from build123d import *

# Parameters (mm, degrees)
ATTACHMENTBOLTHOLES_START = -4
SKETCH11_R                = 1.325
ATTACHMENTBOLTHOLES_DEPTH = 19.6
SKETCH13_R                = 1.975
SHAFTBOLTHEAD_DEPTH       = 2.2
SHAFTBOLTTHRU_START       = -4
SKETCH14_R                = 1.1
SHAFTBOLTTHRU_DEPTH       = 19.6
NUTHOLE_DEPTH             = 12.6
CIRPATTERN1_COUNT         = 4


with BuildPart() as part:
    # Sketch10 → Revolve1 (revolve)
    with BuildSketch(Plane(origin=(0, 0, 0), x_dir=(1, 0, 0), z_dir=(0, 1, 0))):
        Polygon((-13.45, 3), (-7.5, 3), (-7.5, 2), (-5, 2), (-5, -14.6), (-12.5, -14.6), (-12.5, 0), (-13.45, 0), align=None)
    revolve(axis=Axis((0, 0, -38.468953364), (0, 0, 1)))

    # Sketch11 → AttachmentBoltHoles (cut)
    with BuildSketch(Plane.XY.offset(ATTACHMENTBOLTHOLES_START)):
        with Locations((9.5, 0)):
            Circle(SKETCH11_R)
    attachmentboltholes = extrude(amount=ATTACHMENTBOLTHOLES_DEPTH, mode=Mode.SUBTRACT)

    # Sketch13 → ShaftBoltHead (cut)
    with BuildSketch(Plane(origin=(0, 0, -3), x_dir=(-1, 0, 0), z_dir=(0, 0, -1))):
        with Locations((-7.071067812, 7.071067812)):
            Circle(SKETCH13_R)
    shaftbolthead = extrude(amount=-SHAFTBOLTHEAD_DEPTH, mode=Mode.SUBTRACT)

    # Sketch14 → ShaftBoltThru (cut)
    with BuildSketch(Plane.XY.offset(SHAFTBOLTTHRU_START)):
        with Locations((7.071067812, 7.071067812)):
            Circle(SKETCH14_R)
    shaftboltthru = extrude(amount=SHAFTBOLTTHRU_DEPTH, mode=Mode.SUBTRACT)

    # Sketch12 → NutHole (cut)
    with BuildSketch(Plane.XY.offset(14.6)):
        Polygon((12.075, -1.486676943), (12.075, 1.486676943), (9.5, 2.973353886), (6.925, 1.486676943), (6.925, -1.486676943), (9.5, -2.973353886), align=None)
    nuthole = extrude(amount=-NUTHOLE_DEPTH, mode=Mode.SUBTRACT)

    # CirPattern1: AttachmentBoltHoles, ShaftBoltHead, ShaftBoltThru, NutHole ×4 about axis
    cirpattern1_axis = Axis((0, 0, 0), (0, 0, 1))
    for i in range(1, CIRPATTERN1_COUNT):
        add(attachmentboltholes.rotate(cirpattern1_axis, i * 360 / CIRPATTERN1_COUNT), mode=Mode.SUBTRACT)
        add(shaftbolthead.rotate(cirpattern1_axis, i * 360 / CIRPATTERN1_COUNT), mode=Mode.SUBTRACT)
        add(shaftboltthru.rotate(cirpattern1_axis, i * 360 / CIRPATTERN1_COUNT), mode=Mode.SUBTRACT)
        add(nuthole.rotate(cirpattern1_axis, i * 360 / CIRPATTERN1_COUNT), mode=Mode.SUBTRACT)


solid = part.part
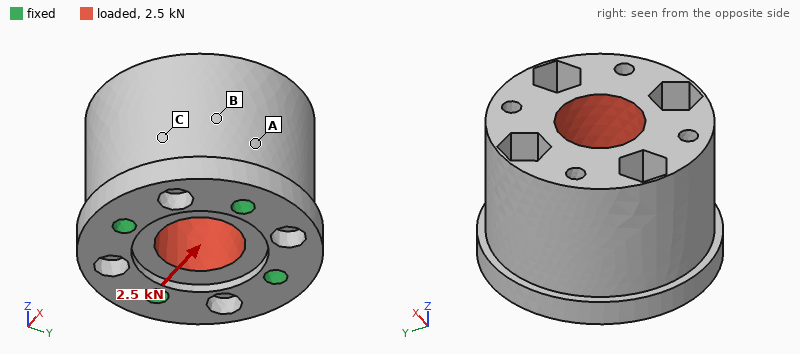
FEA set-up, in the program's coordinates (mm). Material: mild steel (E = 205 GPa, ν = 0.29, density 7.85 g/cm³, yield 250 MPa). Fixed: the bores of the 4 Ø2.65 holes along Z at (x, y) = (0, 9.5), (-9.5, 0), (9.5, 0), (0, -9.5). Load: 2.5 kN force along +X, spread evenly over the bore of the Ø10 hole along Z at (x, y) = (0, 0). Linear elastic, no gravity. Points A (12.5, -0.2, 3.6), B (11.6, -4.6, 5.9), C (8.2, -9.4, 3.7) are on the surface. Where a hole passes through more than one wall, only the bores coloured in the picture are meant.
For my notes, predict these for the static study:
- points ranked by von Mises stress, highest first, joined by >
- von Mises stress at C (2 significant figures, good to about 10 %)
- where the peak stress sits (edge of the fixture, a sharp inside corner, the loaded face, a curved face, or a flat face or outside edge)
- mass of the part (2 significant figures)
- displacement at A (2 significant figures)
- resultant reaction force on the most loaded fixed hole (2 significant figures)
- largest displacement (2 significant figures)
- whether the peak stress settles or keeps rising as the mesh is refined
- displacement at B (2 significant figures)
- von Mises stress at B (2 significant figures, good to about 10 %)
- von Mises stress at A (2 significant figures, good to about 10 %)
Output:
A > B > C
5.3 MPa
edge of the fixture
45 g
0.93 µm
970 N
3.0 µm
keeps rising
1.7 µm
9.6 MPa
25 MPa
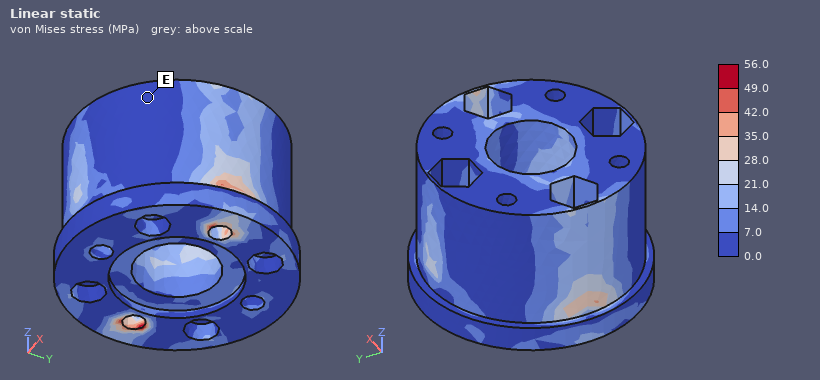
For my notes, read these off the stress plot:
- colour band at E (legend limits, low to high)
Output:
0.0 to 7.0 MPa
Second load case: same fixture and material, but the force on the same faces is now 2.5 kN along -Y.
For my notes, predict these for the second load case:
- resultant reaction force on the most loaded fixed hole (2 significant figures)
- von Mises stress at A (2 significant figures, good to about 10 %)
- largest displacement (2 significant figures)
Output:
970 N
21 MPa
3.0 µm
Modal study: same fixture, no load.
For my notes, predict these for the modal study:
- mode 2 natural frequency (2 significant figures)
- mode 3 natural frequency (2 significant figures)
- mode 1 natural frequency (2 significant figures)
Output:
28 kHz
37 kHz
28 kHz
